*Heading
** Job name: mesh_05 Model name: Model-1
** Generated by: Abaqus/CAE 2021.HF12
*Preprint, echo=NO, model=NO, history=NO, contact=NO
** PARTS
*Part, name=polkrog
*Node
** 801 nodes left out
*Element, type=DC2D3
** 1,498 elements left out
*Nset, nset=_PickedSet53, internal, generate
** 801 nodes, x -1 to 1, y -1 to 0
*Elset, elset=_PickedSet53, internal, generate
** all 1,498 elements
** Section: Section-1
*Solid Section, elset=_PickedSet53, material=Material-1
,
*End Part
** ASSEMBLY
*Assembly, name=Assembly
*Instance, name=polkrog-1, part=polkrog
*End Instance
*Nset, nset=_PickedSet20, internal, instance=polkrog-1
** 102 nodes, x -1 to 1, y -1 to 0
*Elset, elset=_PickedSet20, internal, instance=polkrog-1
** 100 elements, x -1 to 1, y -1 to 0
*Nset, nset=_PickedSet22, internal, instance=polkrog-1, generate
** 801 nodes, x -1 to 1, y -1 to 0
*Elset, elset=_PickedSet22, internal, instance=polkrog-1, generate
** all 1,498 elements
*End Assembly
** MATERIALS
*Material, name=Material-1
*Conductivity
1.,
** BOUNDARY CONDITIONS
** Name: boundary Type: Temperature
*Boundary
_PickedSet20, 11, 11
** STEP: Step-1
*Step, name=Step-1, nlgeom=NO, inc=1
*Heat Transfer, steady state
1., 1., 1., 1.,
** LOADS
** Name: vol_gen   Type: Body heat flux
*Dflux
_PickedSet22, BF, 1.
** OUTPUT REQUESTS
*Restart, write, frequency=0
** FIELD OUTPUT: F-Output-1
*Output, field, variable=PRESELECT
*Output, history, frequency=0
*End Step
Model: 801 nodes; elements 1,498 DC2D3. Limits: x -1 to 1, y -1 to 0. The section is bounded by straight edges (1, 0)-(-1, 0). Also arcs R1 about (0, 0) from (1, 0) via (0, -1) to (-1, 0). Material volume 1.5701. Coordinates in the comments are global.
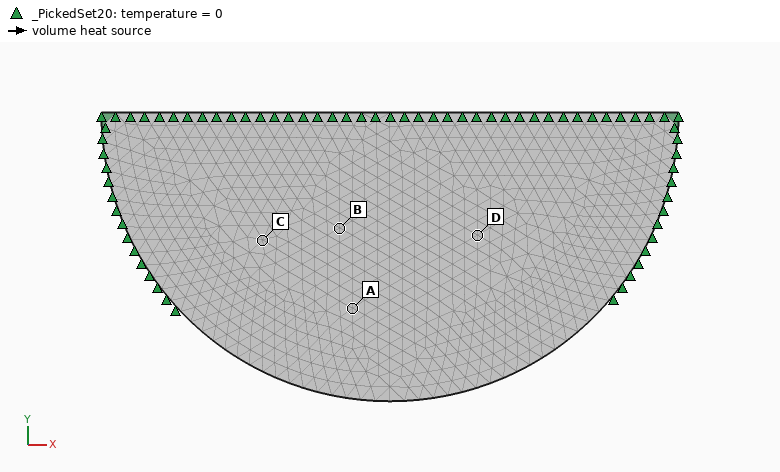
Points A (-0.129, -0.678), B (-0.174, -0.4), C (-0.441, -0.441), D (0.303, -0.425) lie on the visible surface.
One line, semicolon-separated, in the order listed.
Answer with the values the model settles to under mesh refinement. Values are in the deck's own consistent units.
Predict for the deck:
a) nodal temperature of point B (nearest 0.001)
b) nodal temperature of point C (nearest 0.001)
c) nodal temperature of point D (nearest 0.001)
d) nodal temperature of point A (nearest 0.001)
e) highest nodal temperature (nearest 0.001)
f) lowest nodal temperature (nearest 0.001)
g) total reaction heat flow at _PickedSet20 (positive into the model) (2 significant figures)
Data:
0.092; 0.076; 0.087; 0.080; 0.098; 0.000; -1.5
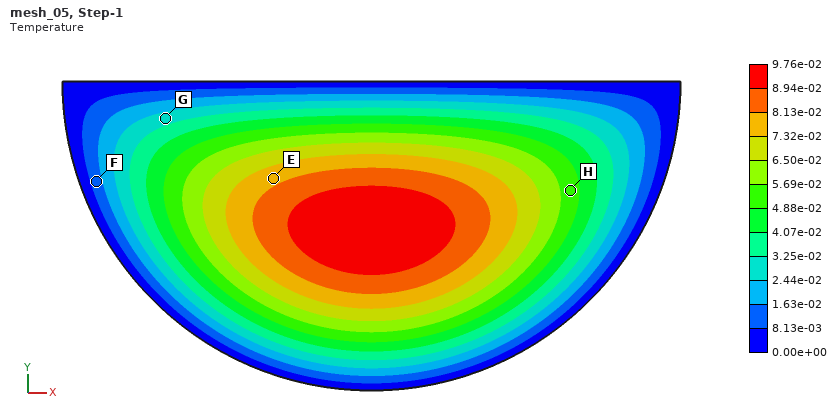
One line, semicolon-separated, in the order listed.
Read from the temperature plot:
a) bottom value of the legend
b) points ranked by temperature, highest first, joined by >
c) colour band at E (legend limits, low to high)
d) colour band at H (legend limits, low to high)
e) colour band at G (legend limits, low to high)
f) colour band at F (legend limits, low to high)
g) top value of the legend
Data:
0.00e+00; E > H > G > F; 7.32e-02 to 8.13e-02; 4.88e-02 to 5.69e-02; 2.44e-02 to 3.25e-02; 8.13e-03 to 1.63e-02; 9.76e-02
